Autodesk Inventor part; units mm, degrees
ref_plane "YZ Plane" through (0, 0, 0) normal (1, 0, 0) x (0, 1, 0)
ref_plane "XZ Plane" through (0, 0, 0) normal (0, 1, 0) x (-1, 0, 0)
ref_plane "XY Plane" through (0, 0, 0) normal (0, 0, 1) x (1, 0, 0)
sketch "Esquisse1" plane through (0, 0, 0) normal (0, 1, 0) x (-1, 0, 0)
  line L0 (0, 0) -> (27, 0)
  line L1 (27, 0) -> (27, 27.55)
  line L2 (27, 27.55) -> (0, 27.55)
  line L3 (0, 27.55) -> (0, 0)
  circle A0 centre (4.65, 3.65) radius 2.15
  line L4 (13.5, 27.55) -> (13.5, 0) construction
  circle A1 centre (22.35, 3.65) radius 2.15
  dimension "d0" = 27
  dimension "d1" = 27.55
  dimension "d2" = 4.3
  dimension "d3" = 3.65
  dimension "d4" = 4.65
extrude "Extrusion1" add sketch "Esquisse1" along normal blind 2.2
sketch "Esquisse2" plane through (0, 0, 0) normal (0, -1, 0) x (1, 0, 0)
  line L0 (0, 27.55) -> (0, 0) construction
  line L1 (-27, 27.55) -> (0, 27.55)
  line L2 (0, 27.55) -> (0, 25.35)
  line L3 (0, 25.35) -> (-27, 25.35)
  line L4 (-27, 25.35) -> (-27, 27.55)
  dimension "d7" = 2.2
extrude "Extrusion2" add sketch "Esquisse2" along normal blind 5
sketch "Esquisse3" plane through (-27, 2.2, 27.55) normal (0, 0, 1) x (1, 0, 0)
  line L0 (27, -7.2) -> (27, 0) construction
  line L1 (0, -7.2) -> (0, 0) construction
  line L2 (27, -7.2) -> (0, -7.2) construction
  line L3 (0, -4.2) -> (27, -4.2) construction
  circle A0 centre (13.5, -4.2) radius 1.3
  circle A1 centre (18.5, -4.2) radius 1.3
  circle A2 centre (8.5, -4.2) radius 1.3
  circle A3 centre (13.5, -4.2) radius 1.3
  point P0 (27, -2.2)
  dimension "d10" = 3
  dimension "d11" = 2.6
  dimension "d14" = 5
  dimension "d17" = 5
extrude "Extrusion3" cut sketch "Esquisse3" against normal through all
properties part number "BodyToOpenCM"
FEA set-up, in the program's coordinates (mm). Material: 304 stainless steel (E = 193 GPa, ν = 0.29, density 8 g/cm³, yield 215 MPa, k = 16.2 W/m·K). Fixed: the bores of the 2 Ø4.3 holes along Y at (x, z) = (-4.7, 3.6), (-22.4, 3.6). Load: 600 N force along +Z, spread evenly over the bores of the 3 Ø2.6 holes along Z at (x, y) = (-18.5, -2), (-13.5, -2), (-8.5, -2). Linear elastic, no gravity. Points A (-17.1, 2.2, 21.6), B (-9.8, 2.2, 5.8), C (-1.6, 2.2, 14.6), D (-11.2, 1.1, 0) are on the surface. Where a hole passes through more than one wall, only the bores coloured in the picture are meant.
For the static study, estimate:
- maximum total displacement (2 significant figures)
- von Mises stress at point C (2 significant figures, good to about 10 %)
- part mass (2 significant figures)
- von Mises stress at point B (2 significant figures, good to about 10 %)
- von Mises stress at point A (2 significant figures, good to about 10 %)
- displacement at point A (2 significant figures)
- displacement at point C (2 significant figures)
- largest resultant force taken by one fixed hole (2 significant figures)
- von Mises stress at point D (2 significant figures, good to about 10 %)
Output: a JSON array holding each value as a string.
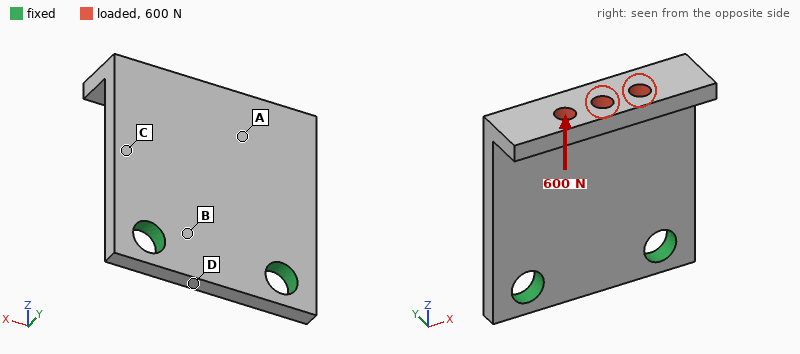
["0.12 mm", "81 MPa", "15 g", "49 MPa", "68 MPa", "0.057 mm", "0.019 mm", "310 N", "14 MPa"]
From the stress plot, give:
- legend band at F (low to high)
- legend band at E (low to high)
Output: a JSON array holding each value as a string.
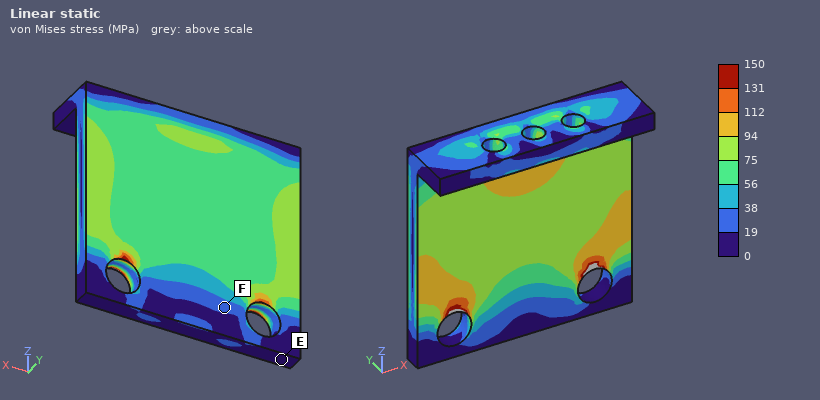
["19 to 38 MPa", "0 to 19 MPa"]
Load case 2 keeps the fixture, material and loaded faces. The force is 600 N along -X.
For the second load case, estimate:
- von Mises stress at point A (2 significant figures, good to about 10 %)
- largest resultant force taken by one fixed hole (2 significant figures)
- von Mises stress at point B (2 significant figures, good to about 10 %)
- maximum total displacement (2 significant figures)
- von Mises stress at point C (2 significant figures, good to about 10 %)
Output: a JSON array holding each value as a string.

["32 MPa", "740 N", "18 MPa", "57 µm", "60 MPa"]
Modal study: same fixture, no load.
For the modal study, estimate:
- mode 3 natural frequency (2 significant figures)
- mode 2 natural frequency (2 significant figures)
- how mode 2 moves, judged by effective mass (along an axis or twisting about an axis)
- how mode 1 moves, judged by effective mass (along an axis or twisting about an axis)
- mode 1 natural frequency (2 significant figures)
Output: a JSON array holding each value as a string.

["15 kHz", "5800 Hz", "twisting about Z", "along Y", "2500 Hz"]
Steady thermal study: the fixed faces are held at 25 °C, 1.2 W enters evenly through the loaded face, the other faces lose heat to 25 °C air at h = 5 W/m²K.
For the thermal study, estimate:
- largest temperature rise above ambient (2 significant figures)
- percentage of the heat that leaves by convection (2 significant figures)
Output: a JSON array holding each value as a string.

["34 K", "11 %"]
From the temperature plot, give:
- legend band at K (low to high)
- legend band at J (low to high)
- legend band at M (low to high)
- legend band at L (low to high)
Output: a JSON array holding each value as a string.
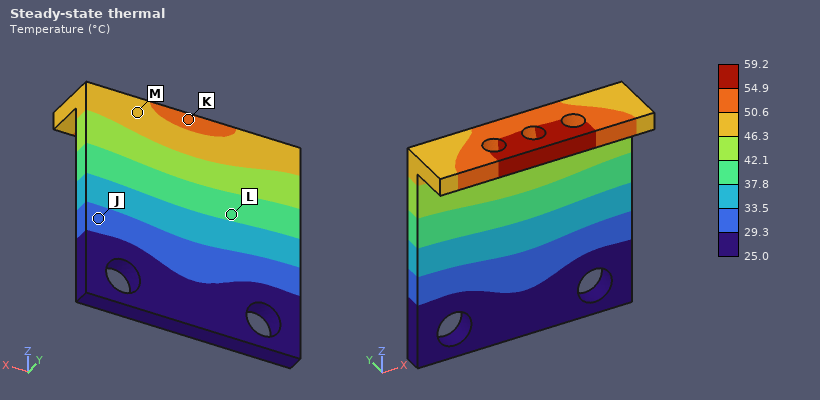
["50.6 to 54.9 °C", "29.3 to 33.5 °C", "46.3 to 50.6 °C", "37.8 to 42.1 °C"]
